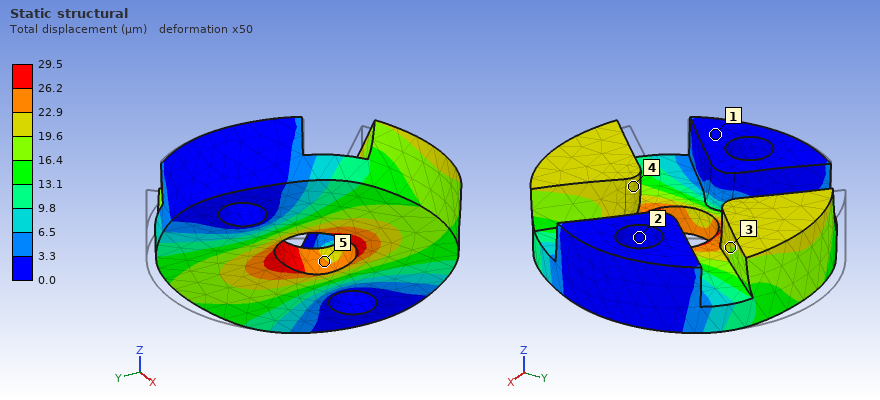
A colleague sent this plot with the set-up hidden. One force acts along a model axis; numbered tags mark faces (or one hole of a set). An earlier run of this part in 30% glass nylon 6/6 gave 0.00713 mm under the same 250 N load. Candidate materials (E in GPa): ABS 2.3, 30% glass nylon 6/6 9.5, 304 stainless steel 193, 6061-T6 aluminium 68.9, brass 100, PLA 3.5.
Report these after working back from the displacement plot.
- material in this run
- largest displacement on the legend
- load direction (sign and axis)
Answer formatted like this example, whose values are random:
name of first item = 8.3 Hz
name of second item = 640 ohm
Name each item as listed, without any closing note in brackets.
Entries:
material in this run = ABS
largest displacement on the legend = 29.5 µm
load direction = -Y
